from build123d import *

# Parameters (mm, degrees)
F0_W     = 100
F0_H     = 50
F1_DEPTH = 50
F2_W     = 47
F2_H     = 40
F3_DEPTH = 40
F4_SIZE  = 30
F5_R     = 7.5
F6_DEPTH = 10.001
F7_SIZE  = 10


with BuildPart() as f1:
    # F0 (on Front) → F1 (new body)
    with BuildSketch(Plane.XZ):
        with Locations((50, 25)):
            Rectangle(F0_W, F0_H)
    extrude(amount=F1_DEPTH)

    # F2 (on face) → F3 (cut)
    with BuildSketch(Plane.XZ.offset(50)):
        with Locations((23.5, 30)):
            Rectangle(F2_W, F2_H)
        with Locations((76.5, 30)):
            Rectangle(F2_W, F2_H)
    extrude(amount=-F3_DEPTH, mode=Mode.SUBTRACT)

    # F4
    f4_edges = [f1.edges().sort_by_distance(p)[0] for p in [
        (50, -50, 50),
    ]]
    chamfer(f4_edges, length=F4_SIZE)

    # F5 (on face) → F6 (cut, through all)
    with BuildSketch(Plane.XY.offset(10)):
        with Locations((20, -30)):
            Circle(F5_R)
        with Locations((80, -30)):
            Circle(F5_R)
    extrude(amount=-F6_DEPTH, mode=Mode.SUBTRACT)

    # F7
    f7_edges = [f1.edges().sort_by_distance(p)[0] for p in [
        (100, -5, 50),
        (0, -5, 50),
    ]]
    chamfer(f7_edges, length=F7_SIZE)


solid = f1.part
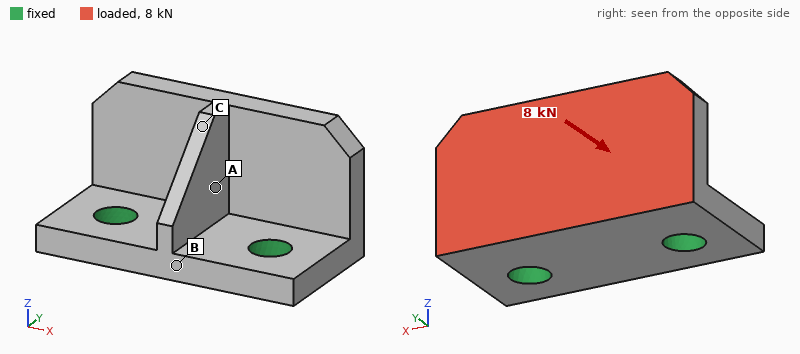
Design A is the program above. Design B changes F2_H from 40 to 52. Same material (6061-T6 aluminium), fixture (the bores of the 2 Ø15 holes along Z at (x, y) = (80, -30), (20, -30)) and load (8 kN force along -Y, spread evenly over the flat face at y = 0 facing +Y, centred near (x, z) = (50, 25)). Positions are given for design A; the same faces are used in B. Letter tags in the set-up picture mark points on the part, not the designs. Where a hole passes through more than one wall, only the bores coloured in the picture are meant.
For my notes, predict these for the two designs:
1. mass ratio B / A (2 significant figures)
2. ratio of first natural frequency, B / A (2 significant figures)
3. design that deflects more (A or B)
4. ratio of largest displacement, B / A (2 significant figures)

0.78
0.34
B
7.8
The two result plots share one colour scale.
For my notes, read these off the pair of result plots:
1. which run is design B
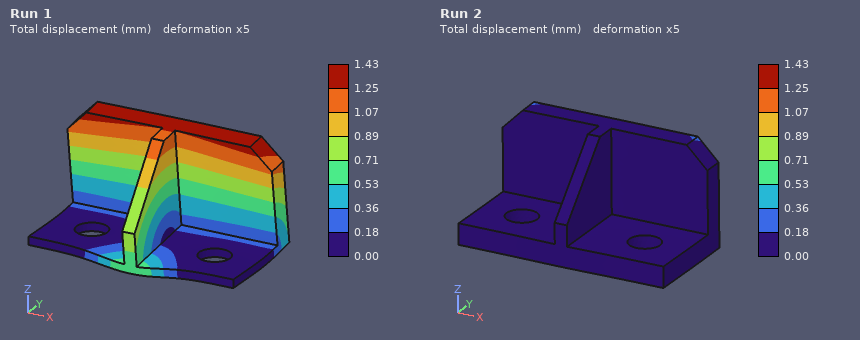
Run 1
